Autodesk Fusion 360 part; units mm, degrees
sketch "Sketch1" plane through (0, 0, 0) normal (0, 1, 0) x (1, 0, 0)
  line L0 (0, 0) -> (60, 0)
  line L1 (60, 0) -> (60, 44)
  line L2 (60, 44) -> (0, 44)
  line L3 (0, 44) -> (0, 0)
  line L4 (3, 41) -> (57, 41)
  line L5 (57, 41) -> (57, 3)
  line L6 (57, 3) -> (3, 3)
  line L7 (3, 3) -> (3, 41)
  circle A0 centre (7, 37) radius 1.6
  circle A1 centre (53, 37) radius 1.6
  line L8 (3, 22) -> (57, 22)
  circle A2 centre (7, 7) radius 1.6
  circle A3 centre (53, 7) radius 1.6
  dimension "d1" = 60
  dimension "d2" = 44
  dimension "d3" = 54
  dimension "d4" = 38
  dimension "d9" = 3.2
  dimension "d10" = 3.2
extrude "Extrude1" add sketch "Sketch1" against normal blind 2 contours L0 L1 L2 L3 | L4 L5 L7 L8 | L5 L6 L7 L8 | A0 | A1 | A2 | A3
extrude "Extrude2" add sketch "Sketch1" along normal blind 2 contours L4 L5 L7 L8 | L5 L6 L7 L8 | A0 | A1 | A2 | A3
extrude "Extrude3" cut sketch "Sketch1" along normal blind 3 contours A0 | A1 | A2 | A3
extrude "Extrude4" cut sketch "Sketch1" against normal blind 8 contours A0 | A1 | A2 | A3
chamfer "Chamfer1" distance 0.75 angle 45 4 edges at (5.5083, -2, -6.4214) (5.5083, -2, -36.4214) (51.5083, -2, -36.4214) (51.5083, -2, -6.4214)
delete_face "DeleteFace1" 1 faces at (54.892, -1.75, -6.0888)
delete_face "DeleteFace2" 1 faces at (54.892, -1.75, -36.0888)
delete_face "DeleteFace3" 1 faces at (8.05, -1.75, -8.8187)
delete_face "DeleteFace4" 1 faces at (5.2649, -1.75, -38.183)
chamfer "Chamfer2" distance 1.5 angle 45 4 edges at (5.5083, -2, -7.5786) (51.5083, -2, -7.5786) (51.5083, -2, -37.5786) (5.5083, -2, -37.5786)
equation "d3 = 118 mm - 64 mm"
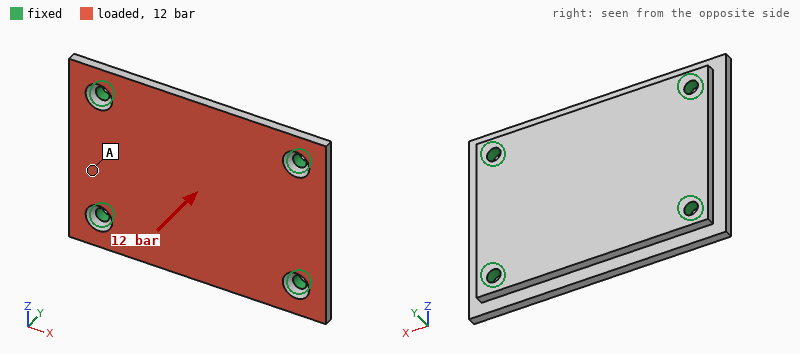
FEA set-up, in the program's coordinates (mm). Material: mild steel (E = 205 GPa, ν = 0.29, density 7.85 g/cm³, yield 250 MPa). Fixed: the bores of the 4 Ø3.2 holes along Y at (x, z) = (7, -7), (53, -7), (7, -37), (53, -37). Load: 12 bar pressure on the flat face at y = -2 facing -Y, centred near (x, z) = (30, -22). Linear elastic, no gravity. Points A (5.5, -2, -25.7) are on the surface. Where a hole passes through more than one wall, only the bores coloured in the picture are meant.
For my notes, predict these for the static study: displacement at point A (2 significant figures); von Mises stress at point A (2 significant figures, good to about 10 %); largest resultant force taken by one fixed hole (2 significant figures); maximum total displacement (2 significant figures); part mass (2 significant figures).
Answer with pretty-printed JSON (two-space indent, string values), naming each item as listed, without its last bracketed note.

{
  "displacement at point A": "4.3 µm",
  "von Mises stress at point A": "28 MPa",
  "largest resultant force taken by one fixed hole": "830 N",
  "maximum total displacement": "25 µm",
  "part mass": "72 g"
}
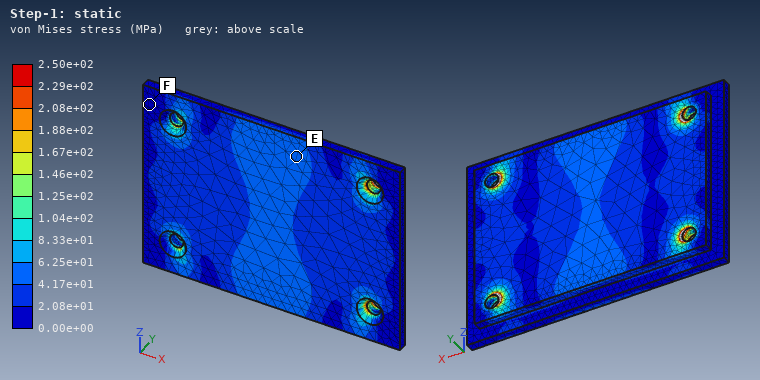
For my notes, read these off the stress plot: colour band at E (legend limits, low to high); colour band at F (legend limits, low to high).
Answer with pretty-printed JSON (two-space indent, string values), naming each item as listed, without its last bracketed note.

{
  "colour band at E": "4.17e+01 to 6.25e+01 MPa",
  "colour band at F": "0.00e+00 to 2.08e+01 MPa"
}
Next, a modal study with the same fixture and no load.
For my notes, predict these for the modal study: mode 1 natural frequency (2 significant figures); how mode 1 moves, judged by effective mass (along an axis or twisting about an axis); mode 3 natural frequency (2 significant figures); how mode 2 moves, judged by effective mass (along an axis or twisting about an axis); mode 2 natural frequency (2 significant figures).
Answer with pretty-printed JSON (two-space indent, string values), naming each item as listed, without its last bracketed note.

{
  "mode 1 natural frequency": "7200 Hz",
  "how mode 1 moves, judged by effective mass": "along Y",
  "mode 3 natural frequency": "16 kHz",
  "how mode 2 moves, judged by effective mass": "twisting about X",
  "mode 2 natural frequency": "10 kHz"
}
